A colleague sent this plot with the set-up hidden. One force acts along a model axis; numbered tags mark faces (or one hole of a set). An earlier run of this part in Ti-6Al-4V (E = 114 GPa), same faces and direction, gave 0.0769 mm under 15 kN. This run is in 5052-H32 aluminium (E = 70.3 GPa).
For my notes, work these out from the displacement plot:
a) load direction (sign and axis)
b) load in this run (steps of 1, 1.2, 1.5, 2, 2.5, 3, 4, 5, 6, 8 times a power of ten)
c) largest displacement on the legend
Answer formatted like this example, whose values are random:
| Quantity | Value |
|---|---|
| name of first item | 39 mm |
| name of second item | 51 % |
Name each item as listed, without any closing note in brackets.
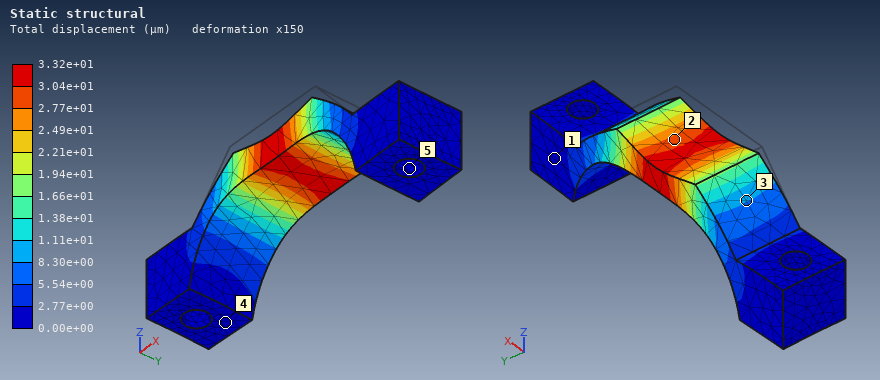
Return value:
| Quantity | Value |
|---|---|
| load direction | -Z |
| load in this run | 4 kN |
| largest displacement on the legend | 3.32e+01 µm |
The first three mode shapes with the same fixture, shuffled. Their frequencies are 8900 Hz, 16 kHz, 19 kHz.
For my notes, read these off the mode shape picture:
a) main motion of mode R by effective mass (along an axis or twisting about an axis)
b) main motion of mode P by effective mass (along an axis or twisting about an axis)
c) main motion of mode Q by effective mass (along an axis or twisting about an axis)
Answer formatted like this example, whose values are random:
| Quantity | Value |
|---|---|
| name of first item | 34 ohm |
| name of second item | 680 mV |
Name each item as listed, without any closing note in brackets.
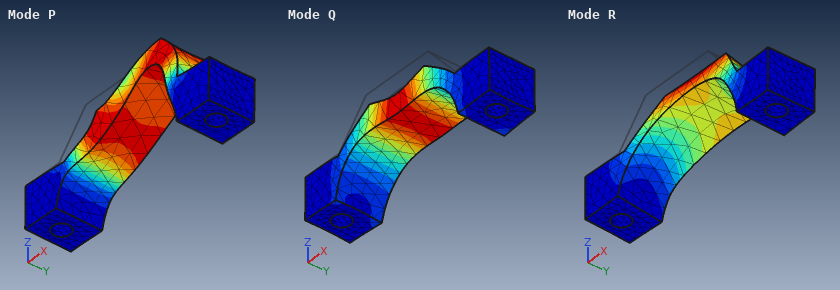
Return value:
| Quantity | Value |
|---|---|
| main motion of mode R by effective mass | along Y |
| main motion of mode P by effective mass | along X |
| main motion of mode Q by effective mass | along Z |
